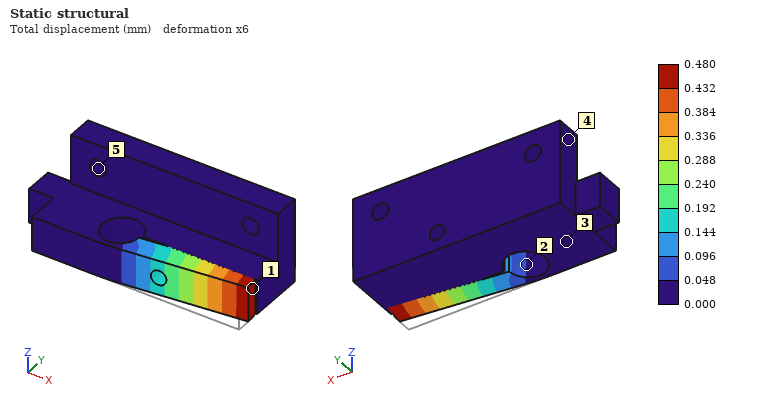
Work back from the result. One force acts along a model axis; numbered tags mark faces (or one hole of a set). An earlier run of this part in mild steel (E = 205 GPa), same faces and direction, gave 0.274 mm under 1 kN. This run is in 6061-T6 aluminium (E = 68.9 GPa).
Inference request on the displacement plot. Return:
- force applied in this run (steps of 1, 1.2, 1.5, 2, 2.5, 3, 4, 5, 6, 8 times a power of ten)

600 N
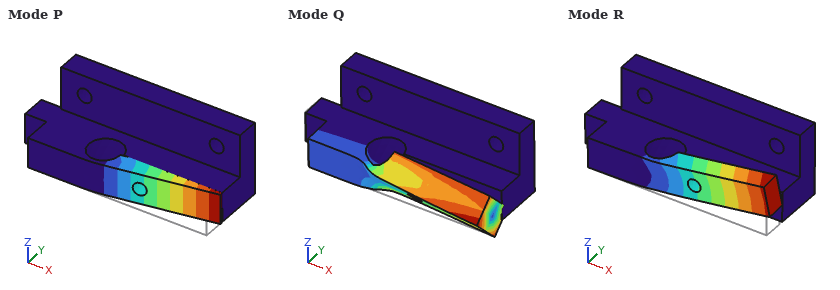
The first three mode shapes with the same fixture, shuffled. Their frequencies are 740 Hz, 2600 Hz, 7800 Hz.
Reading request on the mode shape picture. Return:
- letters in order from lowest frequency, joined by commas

P, R, Q
